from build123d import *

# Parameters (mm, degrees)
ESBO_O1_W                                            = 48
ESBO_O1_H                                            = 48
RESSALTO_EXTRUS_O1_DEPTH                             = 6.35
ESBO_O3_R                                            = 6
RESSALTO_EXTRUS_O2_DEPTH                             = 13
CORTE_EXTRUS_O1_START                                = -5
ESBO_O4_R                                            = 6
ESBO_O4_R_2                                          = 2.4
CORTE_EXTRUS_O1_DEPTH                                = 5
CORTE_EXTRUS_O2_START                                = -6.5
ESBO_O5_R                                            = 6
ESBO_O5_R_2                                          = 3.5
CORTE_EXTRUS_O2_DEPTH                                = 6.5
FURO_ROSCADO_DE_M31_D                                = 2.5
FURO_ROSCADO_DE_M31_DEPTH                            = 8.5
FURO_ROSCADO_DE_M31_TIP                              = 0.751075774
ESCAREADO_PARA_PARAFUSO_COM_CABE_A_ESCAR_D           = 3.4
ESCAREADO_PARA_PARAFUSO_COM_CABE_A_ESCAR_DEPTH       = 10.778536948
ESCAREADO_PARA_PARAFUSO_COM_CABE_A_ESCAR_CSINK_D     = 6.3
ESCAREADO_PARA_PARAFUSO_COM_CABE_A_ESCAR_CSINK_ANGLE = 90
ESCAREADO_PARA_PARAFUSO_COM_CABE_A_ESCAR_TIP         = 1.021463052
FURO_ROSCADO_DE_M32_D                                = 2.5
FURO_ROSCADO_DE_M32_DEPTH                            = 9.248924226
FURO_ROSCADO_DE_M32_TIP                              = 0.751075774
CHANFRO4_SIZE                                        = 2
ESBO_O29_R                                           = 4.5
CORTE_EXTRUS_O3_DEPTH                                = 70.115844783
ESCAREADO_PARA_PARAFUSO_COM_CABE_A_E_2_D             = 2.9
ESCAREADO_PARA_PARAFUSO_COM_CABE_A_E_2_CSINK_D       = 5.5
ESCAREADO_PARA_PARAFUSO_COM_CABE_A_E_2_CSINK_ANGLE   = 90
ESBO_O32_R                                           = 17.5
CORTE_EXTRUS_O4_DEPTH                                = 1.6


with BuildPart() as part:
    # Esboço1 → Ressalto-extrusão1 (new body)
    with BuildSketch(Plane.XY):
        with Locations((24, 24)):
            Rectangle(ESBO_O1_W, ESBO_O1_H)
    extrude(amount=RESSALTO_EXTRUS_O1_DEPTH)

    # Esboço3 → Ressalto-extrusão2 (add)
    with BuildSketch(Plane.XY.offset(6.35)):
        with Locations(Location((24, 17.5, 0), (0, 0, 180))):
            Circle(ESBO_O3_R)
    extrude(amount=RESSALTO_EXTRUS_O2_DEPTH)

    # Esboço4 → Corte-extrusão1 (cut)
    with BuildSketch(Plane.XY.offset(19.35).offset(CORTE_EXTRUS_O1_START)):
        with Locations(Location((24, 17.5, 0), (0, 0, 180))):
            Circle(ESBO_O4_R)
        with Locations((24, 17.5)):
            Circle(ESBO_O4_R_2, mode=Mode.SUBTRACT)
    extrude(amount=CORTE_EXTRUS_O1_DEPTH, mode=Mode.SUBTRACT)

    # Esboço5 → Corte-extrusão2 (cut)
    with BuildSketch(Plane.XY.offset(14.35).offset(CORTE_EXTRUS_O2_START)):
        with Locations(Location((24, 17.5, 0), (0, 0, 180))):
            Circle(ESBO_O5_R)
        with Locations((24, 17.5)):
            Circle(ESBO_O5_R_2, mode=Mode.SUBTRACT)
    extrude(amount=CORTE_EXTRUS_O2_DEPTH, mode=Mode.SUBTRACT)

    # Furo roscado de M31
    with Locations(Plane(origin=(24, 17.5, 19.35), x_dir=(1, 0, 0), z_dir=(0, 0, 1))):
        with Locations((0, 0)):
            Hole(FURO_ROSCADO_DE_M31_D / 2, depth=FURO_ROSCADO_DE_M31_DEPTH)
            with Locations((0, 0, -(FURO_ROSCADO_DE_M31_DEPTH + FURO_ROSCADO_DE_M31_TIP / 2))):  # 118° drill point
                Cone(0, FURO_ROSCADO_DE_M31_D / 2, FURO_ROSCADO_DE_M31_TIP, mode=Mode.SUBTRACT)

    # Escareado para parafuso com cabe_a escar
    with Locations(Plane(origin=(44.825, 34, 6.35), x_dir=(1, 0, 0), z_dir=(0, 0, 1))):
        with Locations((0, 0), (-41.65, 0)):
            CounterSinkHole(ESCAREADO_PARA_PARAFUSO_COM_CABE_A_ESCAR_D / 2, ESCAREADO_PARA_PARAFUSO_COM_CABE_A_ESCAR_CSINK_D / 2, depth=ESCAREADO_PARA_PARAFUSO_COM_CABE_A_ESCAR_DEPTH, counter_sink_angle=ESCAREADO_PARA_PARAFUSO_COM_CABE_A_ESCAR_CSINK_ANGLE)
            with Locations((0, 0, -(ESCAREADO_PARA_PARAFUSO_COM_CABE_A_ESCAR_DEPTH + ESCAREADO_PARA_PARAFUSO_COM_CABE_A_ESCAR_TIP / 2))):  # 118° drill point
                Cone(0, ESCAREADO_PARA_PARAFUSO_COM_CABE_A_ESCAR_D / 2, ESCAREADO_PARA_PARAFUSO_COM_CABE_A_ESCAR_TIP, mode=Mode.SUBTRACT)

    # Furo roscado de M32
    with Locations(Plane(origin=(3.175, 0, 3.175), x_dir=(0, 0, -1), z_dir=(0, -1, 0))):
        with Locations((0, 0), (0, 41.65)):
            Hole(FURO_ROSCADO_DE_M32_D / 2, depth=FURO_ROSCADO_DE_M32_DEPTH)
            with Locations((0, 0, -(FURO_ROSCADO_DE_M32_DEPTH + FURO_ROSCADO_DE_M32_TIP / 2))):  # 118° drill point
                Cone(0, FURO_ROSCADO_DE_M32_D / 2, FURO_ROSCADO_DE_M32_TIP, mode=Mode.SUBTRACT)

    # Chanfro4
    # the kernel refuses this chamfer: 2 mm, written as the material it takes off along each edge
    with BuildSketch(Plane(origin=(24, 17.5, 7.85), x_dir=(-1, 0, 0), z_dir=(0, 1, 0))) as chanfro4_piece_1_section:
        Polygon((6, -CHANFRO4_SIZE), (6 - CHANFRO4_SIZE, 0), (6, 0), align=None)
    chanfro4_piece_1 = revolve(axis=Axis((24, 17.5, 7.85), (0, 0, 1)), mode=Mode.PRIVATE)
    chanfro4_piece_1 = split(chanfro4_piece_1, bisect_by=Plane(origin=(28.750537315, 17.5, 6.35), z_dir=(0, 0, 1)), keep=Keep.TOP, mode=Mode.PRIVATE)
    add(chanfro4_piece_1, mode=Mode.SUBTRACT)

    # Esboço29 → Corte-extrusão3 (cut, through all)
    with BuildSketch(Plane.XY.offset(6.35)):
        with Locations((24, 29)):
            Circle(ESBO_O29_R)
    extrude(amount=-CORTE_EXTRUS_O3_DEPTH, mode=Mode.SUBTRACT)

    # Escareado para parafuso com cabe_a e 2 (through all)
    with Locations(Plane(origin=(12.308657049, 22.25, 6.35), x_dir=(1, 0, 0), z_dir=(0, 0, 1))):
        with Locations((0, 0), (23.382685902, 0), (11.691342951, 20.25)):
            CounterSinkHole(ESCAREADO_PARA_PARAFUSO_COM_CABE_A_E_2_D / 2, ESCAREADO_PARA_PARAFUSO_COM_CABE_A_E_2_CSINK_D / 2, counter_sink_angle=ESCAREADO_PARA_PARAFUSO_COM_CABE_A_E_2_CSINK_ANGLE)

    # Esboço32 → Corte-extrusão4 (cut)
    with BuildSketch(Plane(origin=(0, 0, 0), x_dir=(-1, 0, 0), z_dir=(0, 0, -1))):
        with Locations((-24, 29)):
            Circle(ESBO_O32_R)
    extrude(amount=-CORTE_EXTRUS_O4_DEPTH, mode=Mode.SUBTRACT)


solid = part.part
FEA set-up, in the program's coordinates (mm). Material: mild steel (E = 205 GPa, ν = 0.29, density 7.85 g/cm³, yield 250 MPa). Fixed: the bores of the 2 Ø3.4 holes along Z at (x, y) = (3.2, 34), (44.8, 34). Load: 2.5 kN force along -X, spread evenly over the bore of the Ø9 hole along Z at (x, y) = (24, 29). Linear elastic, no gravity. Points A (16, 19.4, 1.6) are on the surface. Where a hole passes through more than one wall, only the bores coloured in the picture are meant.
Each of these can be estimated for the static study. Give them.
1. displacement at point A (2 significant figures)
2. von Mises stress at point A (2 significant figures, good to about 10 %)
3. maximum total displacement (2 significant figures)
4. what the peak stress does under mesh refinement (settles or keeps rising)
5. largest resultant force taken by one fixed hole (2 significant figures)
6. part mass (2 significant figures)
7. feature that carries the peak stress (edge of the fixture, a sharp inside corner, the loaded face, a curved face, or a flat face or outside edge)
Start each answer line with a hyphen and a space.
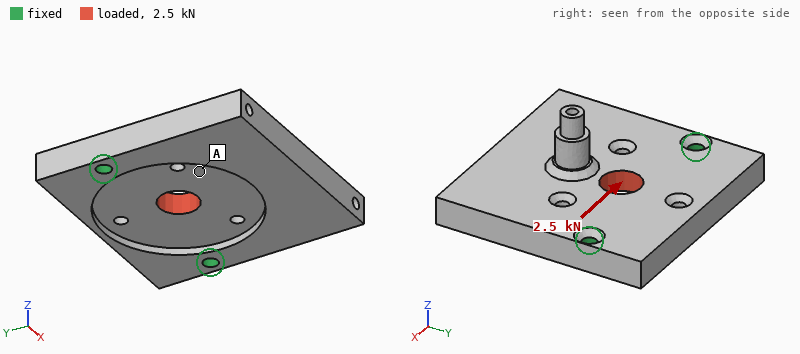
- 1.9 µm
- 5.9 MPa
- 2.6 µm
- keeps rising
- 1.3 kN
- 100 g
- edge of the fixture
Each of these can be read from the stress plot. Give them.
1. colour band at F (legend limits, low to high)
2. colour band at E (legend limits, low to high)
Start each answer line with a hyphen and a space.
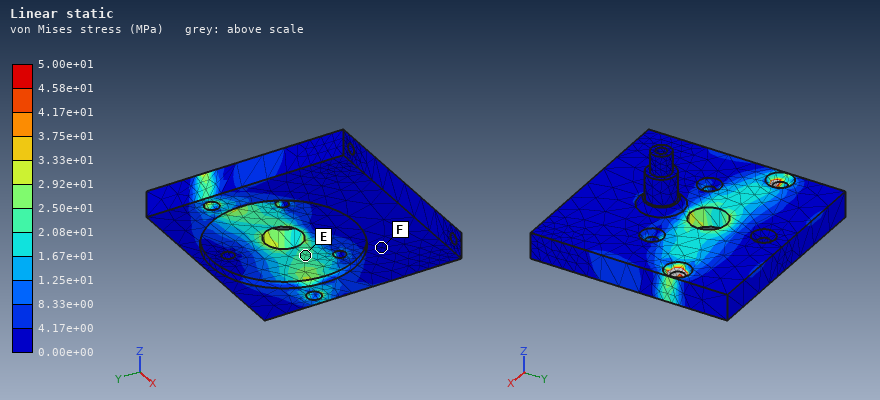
- 0.00e+00 to 4.17e+00 MPa
- 2.08e+01 to 2.50e+01 MPa
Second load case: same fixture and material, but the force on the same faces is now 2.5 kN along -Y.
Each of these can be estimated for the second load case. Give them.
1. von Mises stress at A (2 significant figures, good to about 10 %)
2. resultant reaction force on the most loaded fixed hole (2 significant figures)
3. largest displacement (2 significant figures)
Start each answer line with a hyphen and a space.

- 13 MPa
- 1.3 kN
- 7.4 µm
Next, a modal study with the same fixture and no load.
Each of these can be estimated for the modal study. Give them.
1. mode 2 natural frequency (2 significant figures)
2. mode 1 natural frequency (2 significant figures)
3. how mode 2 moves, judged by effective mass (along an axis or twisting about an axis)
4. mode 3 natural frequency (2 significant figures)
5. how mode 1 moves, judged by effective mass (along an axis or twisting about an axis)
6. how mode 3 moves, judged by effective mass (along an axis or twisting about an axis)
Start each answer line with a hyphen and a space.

- 7100 Hz
- 2800 Hz
- twisting about Y
- 11 kHz
- along Z
- along Z
